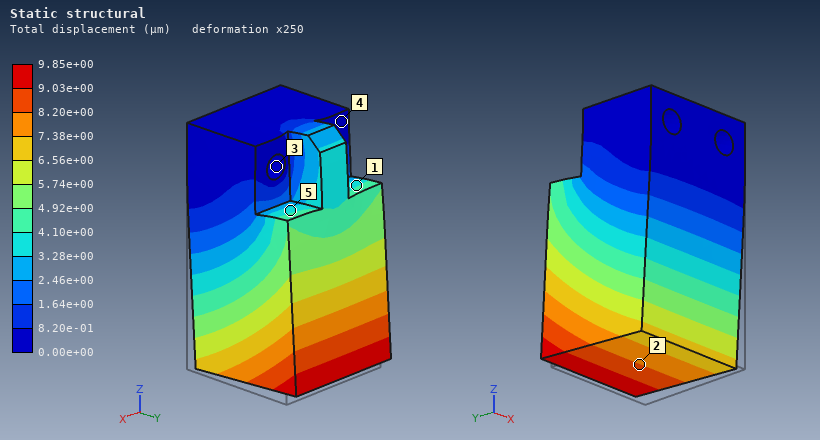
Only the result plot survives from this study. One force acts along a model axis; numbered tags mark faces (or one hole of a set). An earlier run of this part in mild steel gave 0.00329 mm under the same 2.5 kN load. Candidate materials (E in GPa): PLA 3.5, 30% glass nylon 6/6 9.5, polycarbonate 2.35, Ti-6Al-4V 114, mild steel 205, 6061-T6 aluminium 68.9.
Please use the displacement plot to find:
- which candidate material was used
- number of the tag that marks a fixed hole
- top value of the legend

6061-T6 aluminium
3
9.85e+00 µm
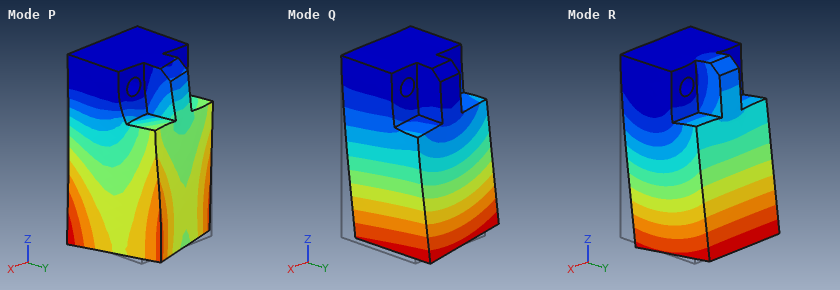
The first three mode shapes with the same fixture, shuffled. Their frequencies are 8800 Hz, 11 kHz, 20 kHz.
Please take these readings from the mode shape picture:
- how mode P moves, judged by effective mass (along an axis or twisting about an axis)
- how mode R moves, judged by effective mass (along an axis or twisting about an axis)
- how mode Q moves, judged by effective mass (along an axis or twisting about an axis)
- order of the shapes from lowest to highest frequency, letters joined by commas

twisting about Z
along Y
along X
R, Q, P
